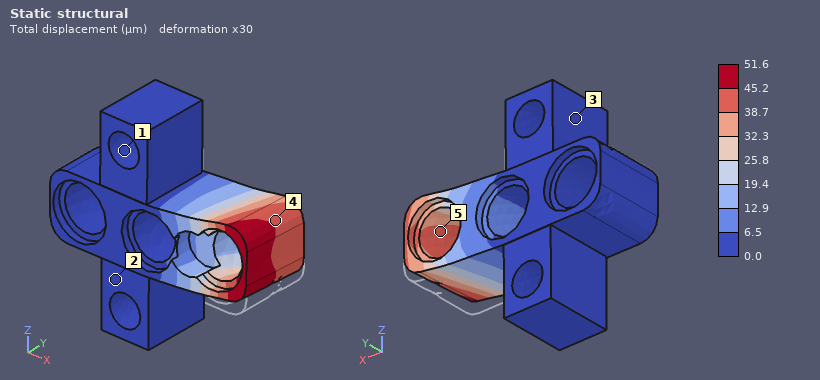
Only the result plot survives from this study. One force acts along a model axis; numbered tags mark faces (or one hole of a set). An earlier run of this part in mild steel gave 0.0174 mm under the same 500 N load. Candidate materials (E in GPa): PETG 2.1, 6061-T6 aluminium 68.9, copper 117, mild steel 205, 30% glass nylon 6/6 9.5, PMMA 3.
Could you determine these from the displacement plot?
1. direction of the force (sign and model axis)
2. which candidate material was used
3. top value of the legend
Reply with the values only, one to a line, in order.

+Z
6061-T6 aluminium
51.6 µm
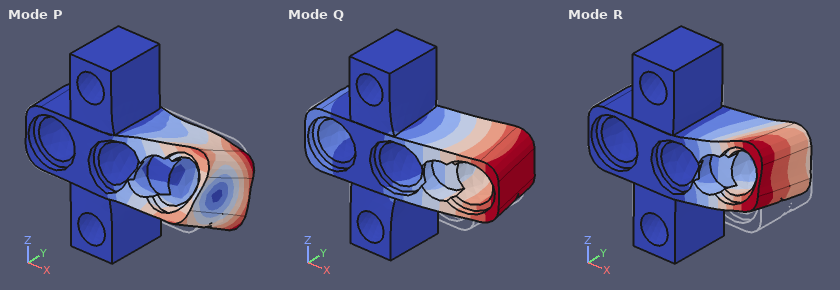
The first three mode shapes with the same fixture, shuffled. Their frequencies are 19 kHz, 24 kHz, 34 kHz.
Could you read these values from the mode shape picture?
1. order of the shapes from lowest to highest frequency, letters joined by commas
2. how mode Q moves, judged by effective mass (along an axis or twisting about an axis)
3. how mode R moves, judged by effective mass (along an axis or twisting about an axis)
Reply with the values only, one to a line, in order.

Q, R, P
along Y
along Z
